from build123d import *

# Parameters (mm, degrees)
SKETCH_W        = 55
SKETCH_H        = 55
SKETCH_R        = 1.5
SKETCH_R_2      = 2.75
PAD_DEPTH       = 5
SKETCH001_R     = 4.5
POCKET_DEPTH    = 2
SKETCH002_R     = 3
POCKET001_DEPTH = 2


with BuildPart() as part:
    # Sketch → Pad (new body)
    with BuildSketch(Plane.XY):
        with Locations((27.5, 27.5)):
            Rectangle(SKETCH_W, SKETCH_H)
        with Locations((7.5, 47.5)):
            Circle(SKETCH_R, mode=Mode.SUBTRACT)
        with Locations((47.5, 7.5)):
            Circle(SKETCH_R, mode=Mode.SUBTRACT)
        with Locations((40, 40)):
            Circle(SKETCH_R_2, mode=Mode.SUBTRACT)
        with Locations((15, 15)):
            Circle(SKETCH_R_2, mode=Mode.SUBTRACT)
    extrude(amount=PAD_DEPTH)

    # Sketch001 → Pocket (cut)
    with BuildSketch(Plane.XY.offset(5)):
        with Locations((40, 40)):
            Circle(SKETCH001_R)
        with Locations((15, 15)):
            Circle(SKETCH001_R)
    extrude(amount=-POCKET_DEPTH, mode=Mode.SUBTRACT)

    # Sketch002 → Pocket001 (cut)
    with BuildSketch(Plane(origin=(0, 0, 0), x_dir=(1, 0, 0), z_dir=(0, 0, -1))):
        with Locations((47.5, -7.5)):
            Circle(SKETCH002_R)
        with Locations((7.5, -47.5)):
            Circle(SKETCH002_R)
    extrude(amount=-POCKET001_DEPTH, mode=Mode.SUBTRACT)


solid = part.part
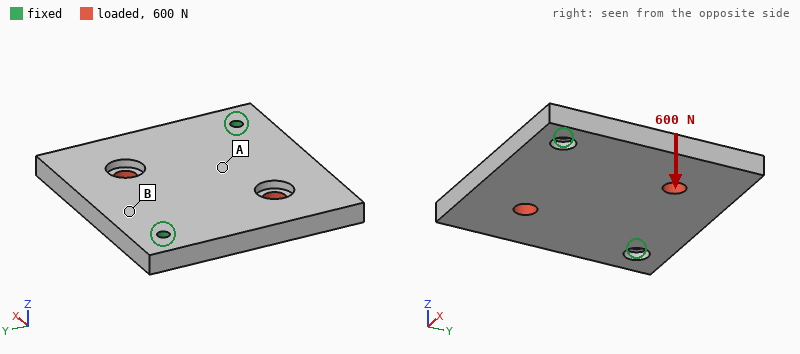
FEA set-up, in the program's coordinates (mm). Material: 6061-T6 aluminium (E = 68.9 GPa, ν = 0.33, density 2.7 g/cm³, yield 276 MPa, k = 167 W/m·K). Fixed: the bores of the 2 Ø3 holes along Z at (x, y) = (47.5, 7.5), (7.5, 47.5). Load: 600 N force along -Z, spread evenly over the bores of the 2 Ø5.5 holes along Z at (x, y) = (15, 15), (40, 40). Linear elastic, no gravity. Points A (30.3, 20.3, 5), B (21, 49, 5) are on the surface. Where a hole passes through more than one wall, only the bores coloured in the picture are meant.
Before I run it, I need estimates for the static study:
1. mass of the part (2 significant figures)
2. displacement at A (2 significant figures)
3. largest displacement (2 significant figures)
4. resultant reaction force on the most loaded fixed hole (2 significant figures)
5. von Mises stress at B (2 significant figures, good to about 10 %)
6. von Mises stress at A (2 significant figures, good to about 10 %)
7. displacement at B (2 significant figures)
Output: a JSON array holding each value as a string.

["39 g", "36 µm", "85 µm", "490 N", "12 MPa", "23 MPa", "22 µm"]
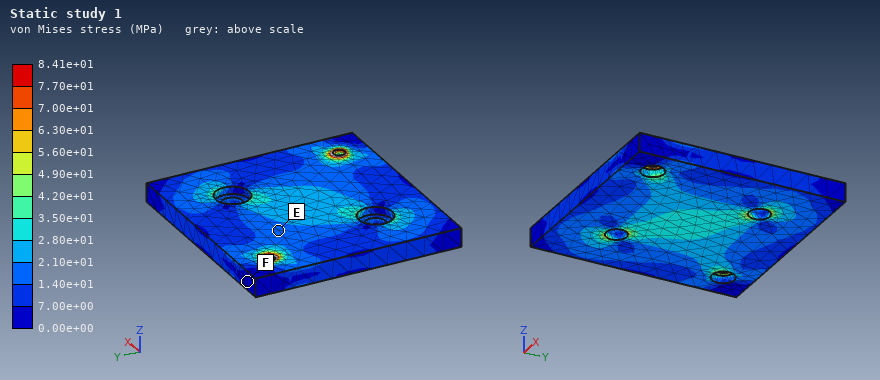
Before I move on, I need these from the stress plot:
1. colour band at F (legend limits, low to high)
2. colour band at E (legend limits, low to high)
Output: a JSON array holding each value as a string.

["0.00e+00 to 7.00e+00 MPa", "1.40e+01 to 2.10e+01 MPa"]
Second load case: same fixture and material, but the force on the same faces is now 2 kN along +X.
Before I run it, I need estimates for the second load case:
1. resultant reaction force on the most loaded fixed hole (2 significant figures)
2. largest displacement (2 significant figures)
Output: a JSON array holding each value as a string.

["1.0 kN", "60 µm"]
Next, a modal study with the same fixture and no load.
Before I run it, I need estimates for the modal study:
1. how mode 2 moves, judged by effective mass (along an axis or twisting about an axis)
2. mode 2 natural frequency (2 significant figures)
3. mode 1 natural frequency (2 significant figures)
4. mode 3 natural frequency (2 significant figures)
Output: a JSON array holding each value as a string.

["along Z", "3400 Hz", "2100 Hz", "9000 Hz"]
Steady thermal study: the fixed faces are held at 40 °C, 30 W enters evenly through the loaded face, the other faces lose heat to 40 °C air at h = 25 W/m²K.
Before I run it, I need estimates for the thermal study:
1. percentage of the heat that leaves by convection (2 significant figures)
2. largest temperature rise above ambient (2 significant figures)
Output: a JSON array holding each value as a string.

["8.0 %", "23 K"]
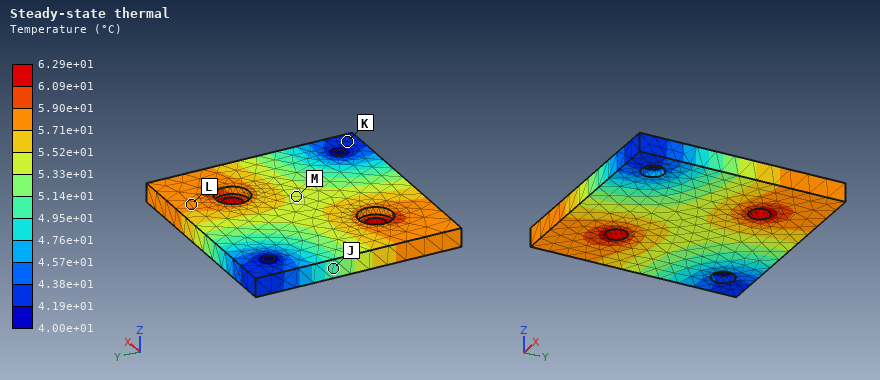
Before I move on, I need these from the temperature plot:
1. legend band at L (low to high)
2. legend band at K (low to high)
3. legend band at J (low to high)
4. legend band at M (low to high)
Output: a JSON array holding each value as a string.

["5.71e+01 to 5.90e+01 °C", "4.19e+01 to 4.38e+01 °C", "4.95e+01 to 5.14e+01 °C", "5.33e+01 to 5.52e+01 °C"]
